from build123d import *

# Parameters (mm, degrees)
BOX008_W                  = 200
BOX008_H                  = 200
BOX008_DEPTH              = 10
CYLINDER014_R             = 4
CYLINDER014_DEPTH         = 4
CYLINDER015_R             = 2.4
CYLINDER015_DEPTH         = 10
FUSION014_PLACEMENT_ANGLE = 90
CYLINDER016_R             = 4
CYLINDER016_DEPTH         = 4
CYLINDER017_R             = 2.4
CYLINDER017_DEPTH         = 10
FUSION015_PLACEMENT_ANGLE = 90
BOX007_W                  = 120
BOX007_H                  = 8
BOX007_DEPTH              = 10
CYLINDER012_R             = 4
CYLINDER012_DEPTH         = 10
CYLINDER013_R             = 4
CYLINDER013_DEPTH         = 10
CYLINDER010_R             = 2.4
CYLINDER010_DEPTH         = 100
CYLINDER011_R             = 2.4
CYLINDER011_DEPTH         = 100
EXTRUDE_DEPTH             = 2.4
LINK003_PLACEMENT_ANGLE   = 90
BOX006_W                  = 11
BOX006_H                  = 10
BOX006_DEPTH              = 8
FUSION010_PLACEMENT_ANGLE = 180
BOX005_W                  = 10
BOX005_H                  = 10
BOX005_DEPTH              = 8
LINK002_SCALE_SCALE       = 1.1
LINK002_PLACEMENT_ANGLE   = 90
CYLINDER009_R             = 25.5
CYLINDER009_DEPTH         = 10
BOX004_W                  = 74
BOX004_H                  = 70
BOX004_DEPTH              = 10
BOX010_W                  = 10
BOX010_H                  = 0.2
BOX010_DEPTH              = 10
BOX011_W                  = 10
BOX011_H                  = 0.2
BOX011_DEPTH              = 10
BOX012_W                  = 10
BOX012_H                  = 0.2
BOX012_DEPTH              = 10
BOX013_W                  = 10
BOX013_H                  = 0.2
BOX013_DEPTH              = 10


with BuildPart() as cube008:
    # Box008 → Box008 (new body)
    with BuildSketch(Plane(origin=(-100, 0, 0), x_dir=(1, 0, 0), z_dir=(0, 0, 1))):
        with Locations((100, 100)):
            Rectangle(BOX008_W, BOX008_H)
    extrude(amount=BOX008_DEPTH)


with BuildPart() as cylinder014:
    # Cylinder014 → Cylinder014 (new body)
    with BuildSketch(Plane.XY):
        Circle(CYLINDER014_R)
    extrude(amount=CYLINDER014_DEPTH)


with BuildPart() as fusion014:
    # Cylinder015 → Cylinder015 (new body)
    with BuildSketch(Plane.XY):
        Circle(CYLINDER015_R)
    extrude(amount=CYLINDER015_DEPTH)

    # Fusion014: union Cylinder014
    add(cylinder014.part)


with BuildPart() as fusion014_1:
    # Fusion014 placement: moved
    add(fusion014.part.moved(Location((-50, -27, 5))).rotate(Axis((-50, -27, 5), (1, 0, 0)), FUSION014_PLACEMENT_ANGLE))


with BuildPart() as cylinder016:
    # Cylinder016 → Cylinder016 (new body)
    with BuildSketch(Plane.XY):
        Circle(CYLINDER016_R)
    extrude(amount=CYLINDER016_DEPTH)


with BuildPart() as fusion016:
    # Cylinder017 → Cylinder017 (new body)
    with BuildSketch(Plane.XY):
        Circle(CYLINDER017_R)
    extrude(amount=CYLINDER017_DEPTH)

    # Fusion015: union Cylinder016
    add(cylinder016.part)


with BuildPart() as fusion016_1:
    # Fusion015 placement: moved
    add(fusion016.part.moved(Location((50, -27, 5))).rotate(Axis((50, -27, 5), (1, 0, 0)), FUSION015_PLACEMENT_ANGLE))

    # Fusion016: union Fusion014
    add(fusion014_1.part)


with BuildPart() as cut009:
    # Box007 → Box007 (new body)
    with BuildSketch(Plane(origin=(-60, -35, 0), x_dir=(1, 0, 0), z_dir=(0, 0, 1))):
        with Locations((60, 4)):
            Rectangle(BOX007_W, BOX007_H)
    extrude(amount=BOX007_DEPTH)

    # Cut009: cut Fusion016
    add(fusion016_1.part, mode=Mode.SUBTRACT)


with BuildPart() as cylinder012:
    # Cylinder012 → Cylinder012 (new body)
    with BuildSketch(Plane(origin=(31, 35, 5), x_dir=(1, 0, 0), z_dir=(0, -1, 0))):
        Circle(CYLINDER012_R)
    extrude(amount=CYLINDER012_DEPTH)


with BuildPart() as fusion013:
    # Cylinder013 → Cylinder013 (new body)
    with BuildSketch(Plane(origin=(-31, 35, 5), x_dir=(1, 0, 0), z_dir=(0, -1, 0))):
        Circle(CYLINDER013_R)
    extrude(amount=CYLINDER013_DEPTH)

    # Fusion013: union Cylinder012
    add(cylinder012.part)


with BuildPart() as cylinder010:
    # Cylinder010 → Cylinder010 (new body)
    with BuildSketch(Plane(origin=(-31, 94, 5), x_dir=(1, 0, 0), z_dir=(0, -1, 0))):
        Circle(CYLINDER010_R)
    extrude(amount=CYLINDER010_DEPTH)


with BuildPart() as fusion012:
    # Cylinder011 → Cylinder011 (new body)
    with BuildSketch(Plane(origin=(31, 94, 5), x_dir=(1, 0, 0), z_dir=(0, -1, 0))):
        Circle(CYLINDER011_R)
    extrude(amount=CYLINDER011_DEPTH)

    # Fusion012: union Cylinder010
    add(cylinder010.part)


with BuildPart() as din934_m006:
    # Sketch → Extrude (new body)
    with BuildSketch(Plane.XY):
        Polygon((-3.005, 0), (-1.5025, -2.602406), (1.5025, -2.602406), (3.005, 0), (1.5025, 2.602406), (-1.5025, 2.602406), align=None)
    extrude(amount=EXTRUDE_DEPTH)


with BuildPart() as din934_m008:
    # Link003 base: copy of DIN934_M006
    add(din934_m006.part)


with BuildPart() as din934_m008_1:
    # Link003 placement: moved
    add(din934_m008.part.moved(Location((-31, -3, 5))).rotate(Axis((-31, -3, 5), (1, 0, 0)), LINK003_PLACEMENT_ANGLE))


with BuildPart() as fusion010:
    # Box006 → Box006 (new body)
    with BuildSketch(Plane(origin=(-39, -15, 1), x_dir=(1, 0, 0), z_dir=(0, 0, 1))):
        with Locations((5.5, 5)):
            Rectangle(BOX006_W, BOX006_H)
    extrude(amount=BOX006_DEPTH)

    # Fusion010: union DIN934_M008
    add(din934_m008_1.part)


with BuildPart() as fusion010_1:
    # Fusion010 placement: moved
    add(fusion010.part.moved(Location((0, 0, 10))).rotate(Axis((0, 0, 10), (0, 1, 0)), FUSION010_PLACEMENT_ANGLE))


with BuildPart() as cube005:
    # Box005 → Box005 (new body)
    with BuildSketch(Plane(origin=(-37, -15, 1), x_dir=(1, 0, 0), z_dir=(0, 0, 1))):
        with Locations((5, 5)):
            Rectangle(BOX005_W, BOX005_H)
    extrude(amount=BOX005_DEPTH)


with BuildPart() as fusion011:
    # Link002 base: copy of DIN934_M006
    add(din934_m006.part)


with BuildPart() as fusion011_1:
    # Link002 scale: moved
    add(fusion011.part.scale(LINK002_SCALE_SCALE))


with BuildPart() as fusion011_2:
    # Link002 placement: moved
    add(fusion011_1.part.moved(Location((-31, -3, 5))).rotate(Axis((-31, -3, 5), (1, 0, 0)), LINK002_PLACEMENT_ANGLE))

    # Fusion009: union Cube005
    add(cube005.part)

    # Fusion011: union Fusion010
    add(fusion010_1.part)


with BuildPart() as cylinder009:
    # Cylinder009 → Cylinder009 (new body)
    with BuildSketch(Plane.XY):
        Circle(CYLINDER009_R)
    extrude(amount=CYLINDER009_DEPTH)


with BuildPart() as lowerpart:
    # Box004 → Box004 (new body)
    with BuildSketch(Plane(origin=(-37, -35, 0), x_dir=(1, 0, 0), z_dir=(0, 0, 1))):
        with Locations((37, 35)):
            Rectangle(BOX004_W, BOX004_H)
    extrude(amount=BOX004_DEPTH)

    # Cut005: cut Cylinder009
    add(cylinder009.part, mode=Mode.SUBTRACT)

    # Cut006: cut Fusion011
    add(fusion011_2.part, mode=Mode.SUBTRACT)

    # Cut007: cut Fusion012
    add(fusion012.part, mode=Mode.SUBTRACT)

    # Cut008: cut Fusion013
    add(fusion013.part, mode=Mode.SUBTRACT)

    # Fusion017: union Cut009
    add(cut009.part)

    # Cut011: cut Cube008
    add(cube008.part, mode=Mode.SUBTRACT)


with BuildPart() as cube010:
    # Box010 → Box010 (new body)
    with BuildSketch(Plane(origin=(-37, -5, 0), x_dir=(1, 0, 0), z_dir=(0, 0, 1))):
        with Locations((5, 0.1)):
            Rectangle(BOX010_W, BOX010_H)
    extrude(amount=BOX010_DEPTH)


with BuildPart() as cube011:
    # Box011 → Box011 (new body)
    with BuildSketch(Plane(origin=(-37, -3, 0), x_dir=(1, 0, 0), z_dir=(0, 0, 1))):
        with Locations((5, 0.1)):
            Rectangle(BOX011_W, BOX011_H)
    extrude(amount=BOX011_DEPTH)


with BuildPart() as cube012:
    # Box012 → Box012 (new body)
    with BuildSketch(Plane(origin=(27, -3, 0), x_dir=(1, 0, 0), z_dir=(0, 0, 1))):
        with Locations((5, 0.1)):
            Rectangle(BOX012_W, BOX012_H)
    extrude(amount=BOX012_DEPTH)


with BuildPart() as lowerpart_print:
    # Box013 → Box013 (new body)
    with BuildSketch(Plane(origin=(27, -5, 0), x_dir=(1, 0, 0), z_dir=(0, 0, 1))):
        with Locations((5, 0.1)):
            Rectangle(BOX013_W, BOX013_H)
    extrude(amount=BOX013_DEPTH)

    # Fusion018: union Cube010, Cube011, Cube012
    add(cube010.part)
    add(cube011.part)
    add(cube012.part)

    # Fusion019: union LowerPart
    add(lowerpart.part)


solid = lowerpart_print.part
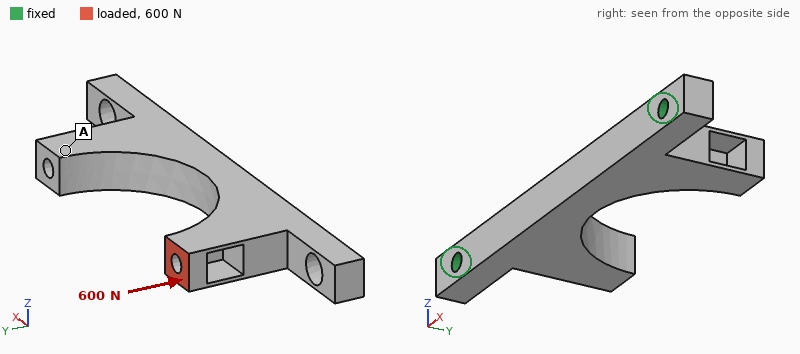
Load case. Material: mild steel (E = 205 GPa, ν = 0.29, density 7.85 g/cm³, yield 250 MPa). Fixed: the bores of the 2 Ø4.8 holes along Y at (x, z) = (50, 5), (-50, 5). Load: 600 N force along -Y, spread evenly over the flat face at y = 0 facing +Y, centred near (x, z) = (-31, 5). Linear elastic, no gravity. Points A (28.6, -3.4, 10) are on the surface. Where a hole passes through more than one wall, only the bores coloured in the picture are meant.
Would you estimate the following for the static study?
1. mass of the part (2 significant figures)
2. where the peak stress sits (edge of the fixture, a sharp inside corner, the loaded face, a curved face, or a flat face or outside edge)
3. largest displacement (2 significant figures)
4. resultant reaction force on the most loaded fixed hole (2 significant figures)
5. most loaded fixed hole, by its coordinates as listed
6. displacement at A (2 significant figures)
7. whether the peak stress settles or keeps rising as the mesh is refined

130 g
edge of the fixture
10 µm
610 N
(-50, 5)
6.9 µm
keeps rising
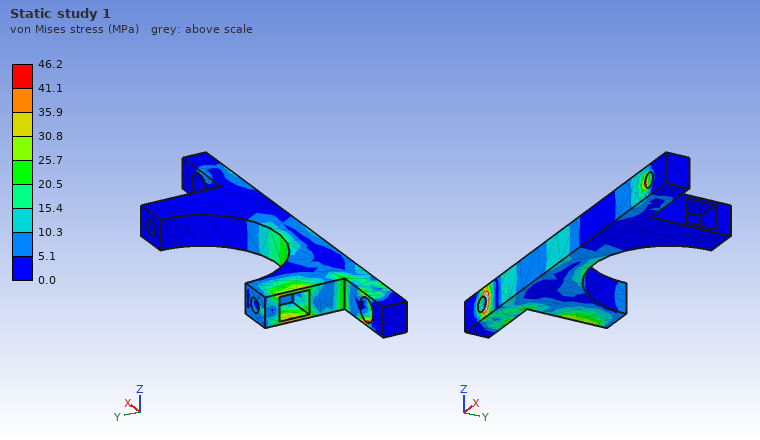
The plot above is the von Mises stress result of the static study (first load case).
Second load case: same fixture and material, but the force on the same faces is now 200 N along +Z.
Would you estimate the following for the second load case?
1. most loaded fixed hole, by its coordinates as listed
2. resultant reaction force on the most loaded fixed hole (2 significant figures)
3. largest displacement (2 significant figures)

(-50, 5)
180 N
53 µm
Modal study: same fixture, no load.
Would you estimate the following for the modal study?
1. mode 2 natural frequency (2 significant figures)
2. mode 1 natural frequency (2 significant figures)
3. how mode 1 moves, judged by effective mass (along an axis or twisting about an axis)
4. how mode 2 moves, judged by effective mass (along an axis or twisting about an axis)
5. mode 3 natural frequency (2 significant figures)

3300 Hz
2700 Hz
along Z
along Y
4500 Hz
